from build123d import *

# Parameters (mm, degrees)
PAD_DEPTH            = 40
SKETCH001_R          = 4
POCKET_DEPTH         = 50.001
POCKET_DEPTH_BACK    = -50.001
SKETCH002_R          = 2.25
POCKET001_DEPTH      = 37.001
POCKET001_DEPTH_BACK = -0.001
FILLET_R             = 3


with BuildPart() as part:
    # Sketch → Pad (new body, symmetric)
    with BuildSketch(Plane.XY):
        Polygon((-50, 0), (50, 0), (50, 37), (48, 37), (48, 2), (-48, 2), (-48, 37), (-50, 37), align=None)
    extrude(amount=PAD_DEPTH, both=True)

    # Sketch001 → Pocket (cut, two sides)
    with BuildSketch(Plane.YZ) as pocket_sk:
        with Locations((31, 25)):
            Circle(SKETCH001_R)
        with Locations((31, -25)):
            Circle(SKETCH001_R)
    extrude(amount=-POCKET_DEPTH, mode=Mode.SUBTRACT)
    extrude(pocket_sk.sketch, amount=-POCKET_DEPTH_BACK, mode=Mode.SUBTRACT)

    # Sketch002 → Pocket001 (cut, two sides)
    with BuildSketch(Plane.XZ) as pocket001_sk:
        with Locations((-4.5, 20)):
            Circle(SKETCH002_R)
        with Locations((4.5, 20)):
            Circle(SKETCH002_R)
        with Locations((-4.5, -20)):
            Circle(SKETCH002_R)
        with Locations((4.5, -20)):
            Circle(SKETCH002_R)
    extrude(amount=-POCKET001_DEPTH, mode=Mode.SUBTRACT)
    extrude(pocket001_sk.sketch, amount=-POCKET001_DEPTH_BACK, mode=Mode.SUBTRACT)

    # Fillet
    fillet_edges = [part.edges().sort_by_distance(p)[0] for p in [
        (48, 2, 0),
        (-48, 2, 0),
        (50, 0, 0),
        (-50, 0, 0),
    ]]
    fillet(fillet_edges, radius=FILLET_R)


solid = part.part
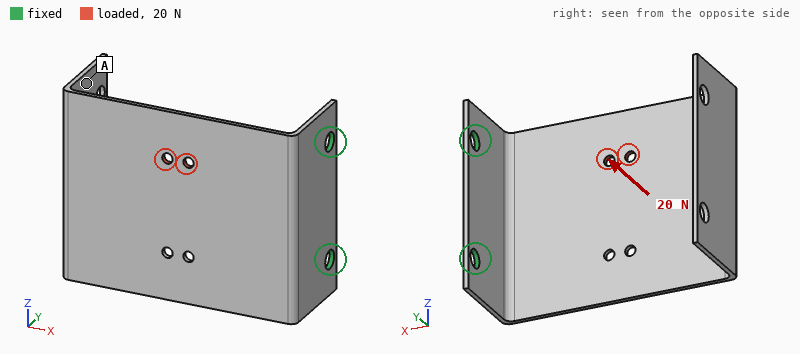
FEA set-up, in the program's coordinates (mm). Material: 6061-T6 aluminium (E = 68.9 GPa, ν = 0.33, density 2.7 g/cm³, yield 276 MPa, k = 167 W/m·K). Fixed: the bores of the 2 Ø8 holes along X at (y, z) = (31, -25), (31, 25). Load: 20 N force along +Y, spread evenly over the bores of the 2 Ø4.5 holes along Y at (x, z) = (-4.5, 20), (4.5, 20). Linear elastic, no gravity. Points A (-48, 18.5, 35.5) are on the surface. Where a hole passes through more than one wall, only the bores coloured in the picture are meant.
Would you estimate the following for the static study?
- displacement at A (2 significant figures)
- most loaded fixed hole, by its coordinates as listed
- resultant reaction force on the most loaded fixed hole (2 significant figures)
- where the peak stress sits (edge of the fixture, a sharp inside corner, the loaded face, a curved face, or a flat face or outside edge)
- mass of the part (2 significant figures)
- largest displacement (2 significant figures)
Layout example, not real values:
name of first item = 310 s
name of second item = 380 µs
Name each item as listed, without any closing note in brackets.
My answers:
displacement at A = 1.2 mm
most loaded fixed hole, by its coordinates as listed = (31, 25)
resultant reaction force on the most loaded fixed hole = 18 N
where the peak stress sits = a flat face or outside edge
mass of the part = 72 g
largest displacement = 1.3 mm
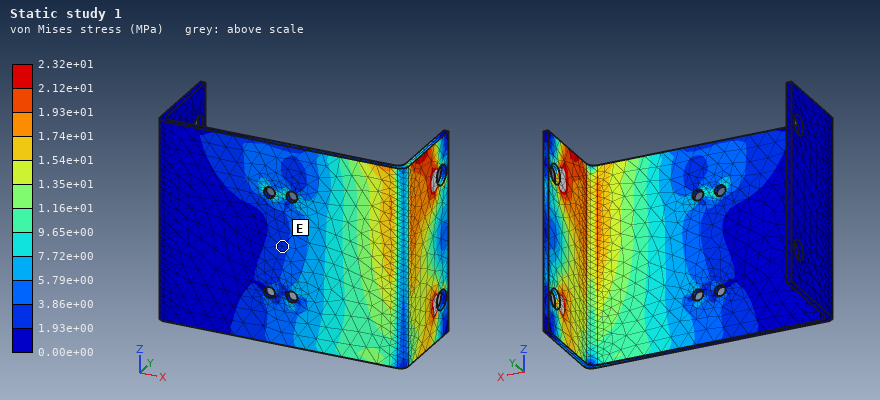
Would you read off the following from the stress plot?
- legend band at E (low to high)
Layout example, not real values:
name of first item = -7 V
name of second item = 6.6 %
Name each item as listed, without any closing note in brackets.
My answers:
legend band at E = 1.93e+00 to 3.86e+00 MPa
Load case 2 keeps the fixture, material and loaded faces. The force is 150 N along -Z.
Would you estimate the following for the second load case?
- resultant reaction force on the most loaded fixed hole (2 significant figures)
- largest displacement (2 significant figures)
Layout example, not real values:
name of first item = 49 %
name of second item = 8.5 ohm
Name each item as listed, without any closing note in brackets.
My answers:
resultant reaction force on the most loaded fixed hole = 170 N
largest displacement = 1.4 mm
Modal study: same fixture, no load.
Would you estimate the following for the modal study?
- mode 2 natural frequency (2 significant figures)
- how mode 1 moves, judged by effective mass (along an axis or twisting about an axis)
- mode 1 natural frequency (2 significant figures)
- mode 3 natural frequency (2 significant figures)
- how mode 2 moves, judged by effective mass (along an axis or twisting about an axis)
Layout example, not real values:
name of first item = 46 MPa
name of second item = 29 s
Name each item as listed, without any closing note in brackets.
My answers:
mode 2 natural frequency = 200 Hz
how mode 1 moves, judged by effective mass = along Y
mode 1 natural frequency = 80 Hz
mode 3 natural frequency = 380 Hz
how mode 2 moves, judged by effective mass = along Z
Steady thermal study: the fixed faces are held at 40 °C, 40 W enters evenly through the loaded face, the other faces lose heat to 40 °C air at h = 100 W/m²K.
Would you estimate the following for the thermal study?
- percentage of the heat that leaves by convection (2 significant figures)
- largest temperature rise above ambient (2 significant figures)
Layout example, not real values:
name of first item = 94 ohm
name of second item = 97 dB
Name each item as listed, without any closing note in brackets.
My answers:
percentage of the heat that leaves by convection = 86 %
largest temperature rise above ambient = 61 K
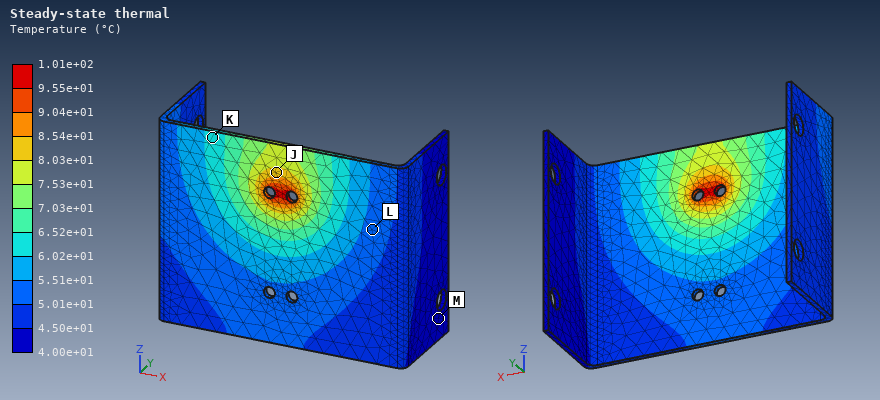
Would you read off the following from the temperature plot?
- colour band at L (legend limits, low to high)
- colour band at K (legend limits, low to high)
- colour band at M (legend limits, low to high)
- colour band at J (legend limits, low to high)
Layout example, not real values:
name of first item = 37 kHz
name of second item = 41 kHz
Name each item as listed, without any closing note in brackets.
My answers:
colour band at L = 5.01e+01 to 5.51e+01 °C
colour band at K = 6.02e+01 to 6.52e+01 °C
colour band at M = 4.00e+01 to 4.50e+01 °C
colour band at J = 8.03e+01 to 8.54e+01 °C
